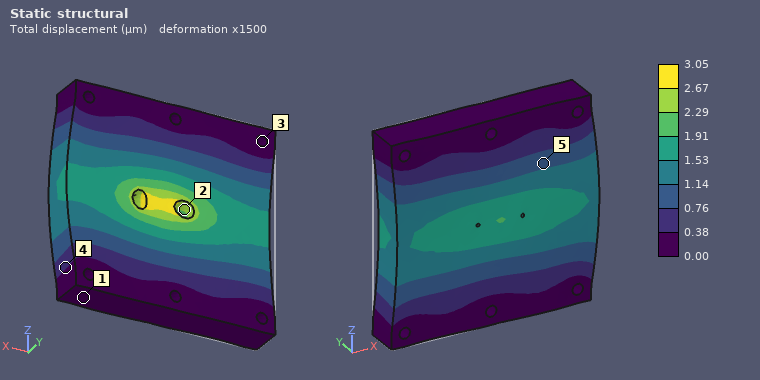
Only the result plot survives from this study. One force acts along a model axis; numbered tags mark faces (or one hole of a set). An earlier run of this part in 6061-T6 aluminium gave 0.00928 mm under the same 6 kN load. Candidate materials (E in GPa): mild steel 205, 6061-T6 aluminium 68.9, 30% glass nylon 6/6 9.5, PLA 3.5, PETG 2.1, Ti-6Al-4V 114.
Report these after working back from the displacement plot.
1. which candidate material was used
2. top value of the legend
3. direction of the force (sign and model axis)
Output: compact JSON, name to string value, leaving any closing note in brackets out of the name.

{"which candidate material was used": "mild steel", "top value of the legend": "3.05 µm", "direction of the force": "+X"}
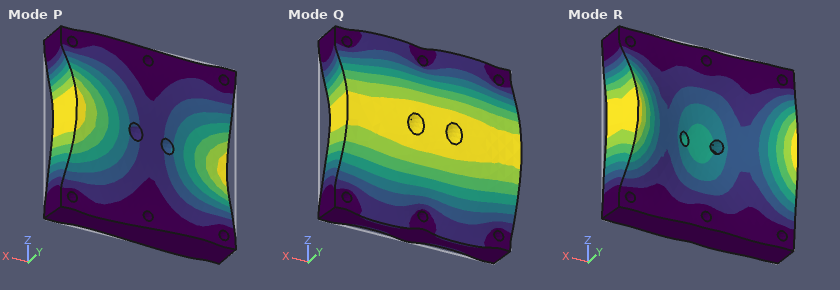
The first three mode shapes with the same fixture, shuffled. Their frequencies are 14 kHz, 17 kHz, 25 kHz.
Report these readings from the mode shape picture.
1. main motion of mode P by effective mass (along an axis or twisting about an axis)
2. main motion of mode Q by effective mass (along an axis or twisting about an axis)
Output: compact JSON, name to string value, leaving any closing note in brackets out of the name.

{"main motion of mode P by effective mass": "twisting about Z", "main motion of mode Q by effective mass": "along Y"}
